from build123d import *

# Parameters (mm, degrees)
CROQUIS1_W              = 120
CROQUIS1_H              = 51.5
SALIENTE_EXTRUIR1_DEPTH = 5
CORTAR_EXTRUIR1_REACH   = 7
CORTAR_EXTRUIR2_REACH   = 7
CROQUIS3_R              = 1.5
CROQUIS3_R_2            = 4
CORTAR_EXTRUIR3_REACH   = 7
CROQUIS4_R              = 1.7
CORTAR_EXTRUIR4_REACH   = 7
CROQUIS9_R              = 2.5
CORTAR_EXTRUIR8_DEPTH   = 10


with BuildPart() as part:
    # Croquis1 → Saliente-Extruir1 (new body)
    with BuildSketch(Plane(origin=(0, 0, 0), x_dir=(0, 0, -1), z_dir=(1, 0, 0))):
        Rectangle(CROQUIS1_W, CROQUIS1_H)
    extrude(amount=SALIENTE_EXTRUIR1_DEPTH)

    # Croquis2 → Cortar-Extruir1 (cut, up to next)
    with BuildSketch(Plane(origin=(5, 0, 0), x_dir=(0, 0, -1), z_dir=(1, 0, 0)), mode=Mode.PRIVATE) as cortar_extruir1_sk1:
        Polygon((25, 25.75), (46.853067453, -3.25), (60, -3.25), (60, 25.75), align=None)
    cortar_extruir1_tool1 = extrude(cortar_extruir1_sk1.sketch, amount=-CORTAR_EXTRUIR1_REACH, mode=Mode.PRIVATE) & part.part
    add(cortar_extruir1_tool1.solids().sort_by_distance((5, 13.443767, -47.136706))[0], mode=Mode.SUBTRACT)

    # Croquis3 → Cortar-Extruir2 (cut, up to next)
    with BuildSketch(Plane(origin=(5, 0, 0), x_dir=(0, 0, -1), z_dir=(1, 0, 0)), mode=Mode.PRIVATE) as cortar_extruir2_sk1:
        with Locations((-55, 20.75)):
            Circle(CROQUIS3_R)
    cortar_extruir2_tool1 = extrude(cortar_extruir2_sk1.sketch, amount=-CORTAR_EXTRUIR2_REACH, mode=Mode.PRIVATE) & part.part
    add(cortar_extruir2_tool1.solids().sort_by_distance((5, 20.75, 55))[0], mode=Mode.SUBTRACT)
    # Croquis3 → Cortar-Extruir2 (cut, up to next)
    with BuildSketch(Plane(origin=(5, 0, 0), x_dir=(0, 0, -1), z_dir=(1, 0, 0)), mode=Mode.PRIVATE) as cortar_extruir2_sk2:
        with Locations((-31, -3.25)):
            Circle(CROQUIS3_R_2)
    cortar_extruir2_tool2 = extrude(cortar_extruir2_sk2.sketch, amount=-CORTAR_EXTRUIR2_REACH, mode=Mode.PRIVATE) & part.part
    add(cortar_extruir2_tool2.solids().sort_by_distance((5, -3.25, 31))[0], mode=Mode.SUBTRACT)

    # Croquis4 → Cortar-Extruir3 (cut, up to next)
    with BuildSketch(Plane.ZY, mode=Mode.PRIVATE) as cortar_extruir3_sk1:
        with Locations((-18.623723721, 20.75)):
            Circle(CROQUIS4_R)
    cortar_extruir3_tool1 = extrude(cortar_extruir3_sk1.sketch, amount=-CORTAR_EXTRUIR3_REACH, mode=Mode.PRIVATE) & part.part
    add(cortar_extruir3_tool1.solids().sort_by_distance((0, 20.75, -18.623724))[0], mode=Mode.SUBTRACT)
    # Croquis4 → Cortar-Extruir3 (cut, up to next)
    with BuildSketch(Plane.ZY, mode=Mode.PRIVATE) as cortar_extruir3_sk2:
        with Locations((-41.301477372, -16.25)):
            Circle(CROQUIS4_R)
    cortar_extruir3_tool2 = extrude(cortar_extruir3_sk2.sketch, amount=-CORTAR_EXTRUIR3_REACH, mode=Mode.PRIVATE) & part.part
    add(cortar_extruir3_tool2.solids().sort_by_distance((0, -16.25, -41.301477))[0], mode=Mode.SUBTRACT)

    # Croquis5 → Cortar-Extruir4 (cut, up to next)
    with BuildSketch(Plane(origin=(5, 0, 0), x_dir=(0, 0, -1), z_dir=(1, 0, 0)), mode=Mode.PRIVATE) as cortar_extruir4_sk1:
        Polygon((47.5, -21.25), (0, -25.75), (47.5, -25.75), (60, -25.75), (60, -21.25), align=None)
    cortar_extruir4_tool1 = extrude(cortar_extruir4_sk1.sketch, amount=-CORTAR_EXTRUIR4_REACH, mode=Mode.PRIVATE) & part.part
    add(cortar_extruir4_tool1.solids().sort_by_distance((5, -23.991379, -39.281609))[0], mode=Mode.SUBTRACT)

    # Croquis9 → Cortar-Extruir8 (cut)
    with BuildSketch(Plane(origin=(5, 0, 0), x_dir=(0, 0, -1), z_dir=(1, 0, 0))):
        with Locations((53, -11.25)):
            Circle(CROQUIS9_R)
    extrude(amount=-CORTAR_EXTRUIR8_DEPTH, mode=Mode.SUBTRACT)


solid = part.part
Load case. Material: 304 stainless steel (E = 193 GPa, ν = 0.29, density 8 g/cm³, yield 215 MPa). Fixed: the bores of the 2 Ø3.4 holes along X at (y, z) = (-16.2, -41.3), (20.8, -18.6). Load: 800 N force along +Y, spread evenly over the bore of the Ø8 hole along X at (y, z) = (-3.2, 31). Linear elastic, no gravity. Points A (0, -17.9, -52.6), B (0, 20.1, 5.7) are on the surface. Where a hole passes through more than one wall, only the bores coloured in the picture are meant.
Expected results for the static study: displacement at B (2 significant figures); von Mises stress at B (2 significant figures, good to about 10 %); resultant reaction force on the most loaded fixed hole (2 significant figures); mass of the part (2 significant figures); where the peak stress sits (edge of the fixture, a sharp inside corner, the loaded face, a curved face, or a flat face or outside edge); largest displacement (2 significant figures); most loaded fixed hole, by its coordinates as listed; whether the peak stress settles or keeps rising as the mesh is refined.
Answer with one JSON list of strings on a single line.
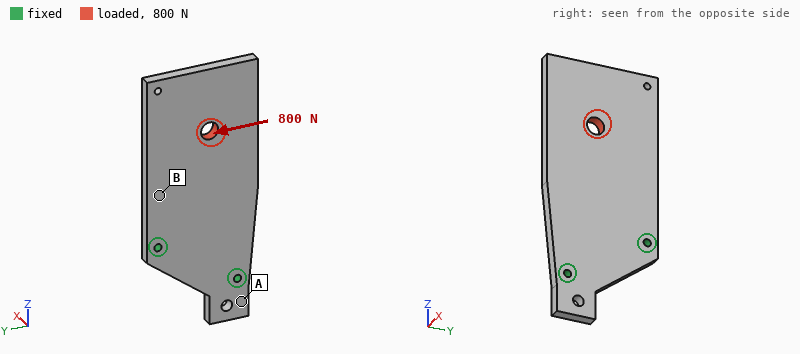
["4.3 µm", "8.2 MPa", "1.3 kN", "210 g", "edge of the fixture", "14 µm", "(20.8, -18.6)", "keeps rising"]
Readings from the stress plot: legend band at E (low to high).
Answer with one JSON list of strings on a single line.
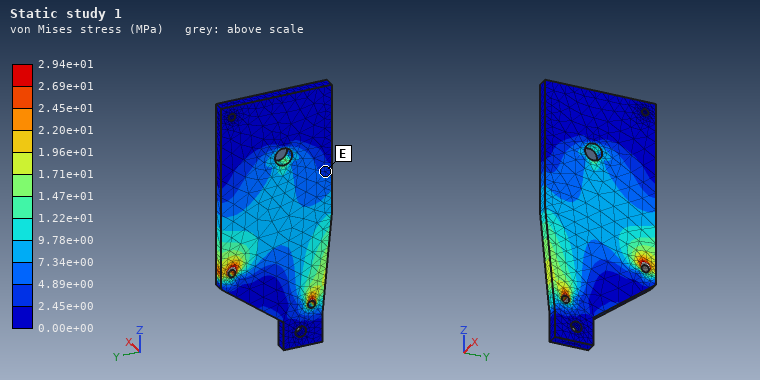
["2.45e+00 to 4.89e+00 MPa"]
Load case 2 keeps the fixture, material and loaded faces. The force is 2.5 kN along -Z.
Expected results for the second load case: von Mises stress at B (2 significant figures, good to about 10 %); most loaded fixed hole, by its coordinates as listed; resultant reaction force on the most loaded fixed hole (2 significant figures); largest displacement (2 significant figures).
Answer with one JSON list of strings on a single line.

["6.4 MPa", "(-16.2, -41.3)", "1.6 kN", "9.5 µm"]
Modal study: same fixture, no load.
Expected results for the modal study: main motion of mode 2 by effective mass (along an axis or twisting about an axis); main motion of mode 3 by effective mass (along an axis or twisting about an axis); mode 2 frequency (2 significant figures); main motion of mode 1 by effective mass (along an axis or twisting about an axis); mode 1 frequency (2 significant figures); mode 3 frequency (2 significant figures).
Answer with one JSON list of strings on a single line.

["twisting about Z", "along X", "1800 Hz", "along X", "510 Hz", "3000 Hz"]
